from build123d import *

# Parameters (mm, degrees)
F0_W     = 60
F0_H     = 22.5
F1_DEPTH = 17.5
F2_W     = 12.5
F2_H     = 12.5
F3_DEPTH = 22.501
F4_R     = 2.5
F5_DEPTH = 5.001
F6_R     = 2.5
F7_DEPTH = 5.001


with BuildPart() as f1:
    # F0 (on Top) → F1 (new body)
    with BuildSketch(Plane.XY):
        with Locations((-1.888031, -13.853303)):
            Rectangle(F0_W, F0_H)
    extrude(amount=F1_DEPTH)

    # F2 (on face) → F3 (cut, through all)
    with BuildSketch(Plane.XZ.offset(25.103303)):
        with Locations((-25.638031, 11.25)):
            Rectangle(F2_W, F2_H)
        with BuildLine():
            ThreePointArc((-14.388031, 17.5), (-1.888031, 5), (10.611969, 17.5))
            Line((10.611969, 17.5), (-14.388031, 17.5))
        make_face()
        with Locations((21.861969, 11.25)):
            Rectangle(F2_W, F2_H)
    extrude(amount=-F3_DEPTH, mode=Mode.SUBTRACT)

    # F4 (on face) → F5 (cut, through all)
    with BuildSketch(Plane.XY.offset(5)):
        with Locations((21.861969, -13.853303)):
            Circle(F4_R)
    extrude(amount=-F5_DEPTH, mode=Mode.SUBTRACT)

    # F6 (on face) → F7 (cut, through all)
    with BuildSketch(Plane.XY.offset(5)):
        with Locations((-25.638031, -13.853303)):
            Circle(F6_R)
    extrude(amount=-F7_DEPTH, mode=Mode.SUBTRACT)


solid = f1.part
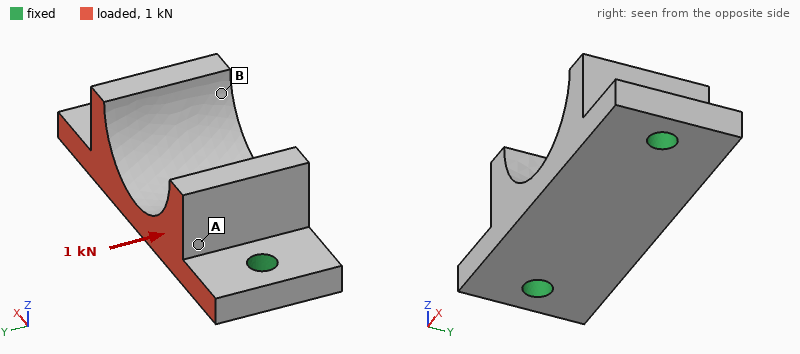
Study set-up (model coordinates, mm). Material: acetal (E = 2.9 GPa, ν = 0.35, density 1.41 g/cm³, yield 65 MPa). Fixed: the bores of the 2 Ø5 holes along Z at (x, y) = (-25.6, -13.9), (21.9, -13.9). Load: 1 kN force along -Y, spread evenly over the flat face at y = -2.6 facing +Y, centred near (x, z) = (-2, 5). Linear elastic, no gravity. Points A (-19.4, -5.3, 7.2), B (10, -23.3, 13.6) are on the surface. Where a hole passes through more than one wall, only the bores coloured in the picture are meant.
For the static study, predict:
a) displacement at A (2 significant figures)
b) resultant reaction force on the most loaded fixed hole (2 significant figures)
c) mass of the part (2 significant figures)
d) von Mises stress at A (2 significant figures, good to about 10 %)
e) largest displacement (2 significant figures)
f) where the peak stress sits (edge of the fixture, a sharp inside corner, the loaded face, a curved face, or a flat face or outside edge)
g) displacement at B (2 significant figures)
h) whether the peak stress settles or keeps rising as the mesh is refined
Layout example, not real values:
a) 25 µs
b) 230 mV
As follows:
a) 0.12 mm
b) 500 N
c) 15 g
d) 5.9 MPa
e) 0.24 mm
f) edge of the fixture
g) 0.19 mm
h) keeps rising
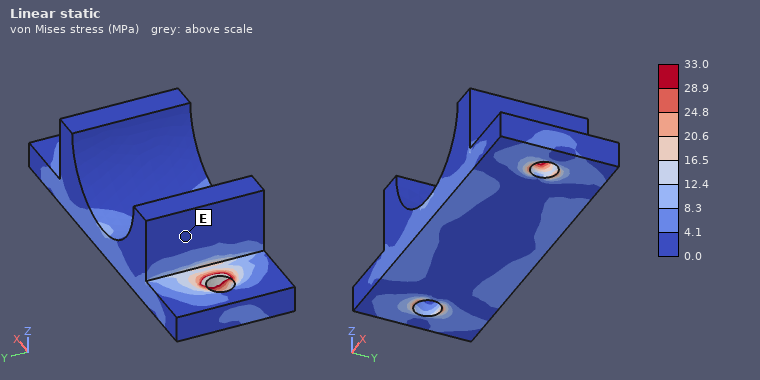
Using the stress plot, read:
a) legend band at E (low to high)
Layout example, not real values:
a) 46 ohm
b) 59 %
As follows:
a) 0.0 to 4.1 MPa
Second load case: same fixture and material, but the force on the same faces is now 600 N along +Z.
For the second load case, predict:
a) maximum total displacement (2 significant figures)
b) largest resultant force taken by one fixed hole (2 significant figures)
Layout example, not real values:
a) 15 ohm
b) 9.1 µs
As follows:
a) 0.49 mm
b) 310 N
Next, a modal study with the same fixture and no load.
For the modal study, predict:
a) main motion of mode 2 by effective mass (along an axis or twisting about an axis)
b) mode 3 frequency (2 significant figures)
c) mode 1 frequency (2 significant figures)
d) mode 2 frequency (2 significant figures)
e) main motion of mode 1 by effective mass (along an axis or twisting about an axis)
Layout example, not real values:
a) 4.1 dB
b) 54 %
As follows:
a) along Y
b) 4500 Hz
c) 2400 Hz
d) 2700 Hz
e) along Z
